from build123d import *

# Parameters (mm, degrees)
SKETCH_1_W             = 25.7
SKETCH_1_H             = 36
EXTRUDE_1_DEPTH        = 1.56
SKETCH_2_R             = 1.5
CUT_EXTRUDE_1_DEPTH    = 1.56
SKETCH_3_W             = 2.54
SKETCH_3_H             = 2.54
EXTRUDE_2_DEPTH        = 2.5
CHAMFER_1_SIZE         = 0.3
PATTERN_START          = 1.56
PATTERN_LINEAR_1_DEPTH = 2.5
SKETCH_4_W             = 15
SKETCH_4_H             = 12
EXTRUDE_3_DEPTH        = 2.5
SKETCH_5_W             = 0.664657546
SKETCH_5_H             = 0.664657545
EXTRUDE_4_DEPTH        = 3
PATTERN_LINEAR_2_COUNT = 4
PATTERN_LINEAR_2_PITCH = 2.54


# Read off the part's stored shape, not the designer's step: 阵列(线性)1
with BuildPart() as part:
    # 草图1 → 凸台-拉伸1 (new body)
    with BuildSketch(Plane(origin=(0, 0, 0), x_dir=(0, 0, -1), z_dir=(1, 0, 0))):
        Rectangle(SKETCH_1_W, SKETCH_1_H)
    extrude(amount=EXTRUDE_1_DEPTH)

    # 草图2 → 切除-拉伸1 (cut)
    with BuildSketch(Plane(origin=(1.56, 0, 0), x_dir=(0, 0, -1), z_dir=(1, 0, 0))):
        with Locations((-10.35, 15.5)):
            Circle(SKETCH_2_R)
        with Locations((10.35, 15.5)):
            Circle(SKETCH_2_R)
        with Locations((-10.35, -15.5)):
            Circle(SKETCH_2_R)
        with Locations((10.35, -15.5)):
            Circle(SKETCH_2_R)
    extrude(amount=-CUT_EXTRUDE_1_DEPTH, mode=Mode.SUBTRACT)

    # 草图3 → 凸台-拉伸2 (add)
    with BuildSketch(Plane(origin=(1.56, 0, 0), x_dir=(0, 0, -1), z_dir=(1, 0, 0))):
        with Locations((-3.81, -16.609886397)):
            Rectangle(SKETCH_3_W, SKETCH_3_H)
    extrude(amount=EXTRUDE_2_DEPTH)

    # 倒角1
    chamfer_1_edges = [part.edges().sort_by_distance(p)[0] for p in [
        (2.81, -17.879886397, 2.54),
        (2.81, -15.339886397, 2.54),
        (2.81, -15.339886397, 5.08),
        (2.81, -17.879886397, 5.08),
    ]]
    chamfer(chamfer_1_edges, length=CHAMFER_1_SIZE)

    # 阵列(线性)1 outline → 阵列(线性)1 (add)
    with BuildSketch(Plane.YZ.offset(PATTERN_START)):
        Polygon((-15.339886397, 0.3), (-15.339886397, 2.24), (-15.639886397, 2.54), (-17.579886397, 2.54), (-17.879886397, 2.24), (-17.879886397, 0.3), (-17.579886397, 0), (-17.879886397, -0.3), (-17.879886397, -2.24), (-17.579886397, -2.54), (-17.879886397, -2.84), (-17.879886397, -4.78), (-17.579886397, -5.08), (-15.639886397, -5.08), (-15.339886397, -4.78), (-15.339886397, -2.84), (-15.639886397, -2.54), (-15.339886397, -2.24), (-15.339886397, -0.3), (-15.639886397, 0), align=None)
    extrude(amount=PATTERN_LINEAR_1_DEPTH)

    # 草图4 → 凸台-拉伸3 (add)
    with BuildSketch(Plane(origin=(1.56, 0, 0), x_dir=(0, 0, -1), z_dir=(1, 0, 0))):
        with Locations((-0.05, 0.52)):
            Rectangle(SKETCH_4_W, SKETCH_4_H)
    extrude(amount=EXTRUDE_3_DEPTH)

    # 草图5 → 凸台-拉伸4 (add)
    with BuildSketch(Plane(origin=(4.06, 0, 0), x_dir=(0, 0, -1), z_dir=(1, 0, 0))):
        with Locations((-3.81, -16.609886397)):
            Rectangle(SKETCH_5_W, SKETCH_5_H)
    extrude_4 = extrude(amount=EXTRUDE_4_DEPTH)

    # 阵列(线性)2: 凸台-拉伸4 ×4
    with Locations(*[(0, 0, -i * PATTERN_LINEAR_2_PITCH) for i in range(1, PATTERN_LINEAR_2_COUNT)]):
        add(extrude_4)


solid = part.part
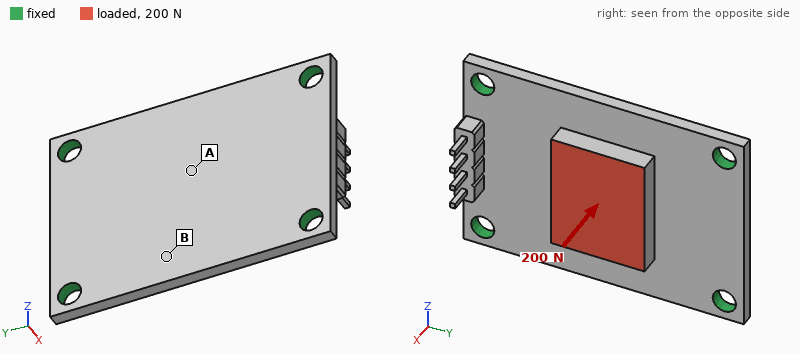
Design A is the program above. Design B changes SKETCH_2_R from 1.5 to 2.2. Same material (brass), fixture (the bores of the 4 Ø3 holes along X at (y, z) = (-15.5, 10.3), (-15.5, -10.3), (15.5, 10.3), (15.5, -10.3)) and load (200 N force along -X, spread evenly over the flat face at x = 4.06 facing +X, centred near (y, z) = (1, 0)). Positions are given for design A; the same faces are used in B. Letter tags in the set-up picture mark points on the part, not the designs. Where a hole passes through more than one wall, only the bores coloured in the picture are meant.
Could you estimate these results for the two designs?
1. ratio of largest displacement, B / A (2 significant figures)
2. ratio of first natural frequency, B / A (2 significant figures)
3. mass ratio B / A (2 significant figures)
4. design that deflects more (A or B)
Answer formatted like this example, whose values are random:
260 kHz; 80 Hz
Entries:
0.80; 1.1; 0.97; A
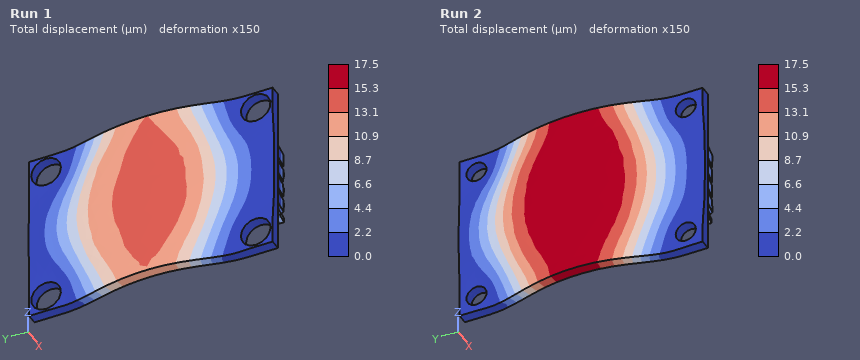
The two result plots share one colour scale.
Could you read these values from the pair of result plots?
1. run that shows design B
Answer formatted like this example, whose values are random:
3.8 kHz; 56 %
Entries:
Run 1
